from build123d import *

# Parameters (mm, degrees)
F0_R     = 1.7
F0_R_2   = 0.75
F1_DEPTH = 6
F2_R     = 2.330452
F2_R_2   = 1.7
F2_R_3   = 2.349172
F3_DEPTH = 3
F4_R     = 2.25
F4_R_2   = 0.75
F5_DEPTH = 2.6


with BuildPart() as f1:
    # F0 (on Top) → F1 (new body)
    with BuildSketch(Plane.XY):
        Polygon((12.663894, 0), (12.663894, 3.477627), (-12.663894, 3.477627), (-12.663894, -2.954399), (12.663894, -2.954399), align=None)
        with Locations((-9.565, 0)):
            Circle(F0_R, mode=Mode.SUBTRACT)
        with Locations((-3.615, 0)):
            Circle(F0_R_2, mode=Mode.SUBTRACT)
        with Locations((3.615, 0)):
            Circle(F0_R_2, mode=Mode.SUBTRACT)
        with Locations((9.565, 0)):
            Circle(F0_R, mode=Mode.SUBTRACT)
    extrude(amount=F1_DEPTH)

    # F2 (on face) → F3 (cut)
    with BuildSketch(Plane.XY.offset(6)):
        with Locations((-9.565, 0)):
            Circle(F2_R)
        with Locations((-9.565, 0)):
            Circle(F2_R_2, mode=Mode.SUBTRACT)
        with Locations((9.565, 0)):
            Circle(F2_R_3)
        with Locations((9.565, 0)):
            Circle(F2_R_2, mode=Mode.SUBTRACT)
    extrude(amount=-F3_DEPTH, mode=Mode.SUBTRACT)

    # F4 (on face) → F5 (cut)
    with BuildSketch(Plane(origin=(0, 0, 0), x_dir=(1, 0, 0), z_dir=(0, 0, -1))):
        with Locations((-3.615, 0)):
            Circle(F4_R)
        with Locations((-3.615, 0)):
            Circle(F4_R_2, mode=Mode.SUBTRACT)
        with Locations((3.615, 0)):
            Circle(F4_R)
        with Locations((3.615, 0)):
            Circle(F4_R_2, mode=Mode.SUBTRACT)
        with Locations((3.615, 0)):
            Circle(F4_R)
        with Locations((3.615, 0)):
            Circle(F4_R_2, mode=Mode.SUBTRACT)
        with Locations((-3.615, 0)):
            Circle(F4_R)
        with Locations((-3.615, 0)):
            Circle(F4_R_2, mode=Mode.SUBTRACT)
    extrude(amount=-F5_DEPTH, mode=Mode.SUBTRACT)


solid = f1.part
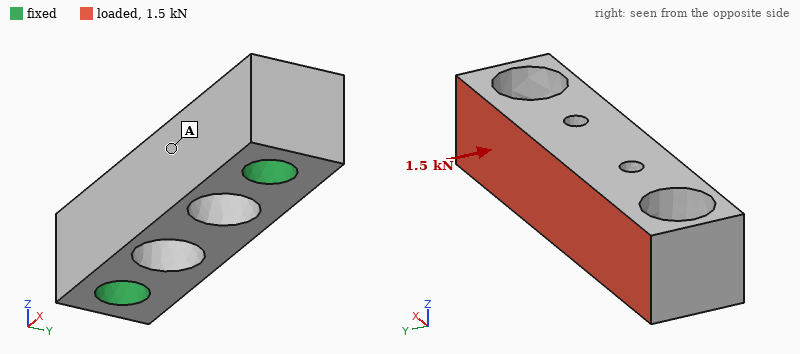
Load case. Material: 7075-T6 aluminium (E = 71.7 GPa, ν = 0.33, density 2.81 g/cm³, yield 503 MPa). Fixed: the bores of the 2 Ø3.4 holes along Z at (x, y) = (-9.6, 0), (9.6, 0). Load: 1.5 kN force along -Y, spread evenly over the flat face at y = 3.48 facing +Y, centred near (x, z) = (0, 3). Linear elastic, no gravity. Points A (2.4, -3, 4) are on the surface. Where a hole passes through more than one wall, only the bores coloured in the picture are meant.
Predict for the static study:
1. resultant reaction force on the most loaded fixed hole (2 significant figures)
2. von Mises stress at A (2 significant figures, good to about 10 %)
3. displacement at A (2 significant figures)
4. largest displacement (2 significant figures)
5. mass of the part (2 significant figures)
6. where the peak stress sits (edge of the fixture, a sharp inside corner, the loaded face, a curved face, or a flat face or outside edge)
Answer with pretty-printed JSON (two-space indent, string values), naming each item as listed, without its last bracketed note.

{
  "resultant reaction force on the most loaded fixed hole": "750 N",
  "von Mises stress at A": "36 MPa",
  "displacement at A": "8.6 µm",
  "largest displacement": "11 µm",
  "mass of the part": "2.0 g",
  "where the peak stress sits": "edge of the fixture"
}
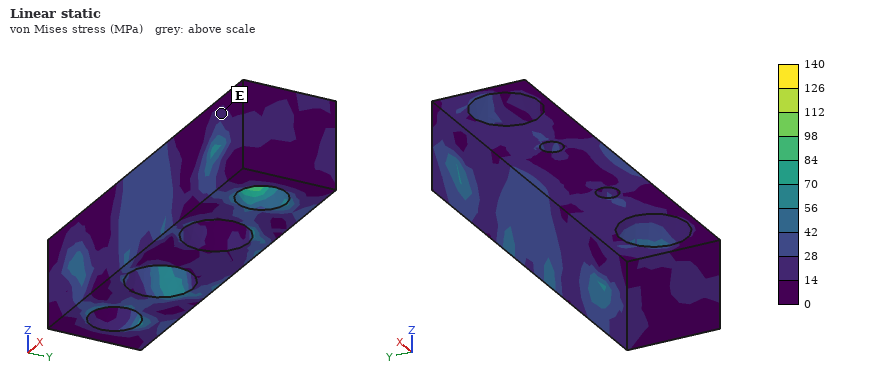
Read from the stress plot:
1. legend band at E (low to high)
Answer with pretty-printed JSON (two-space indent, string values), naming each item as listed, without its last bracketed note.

{
  "legend band at E": "14 to 28 MPa"
}
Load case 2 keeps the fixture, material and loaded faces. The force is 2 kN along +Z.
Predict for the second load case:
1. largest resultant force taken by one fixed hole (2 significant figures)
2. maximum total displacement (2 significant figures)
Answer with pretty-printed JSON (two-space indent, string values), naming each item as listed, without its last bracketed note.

{
  "largest resultant force taken by one fixed hole": "1.0 kN",
  "maximum total displacement": "28 µm"
}
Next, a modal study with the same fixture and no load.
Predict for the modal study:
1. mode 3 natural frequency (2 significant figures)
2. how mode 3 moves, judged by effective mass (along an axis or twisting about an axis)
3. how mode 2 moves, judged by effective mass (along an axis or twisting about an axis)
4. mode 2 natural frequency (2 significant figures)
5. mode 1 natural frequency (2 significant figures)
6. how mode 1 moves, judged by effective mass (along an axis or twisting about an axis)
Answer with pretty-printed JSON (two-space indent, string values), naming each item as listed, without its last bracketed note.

{
  "mode 3 natural frequency": "57 kHz",
  "how mode 3 moves, judged by effective mass": "twisting about X",
  "how mode 2 moves, judged by effective mass": "along Z",
  "mode 2 natural frequency": "53 kHz",
  "mode 1 natural frequency": "46 kHz",
  "how mode 1 moves, judged by effective mass": "along Y"
}
